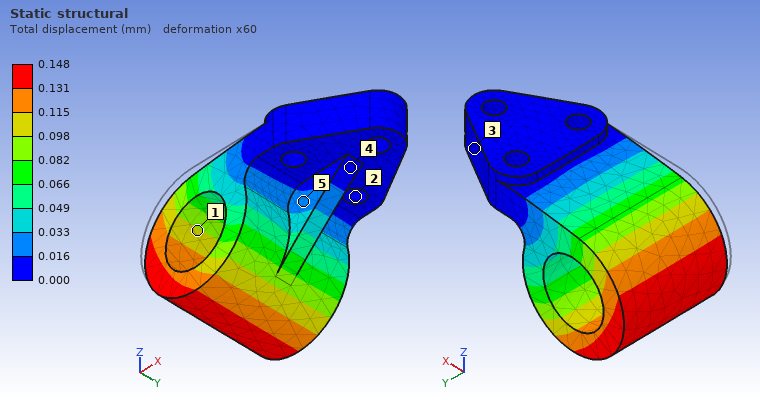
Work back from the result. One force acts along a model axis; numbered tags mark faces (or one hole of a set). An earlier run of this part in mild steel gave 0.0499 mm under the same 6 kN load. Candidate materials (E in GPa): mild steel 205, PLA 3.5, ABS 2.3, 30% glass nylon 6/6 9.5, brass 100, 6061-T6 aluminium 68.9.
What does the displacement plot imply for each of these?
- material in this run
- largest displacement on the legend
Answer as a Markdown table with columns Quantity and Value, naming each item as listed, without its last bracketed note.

| Quantity | Value |
|---|---|
| material in this run | 6061-T6 aluminium |
| largest displacement on the legend | 0.148 mm |
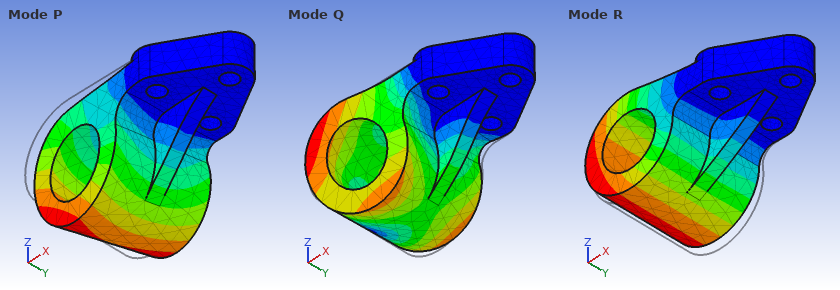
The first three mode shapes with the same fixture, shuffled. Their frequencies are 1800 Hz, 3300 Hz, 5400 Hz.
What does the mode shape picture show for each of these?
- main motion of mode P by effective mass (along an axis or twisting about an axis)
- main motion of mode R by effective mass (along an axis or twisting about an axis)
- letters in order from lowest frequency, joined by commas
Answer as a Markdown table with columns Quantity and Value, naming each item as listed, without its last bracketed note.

| Quantity | Value |
|---|---|
| main motion of mode P by effective mass | along Y |
| main motion of mode R by effective mass | along Z |
| letters in order from lowest frequency, joined by commas | R, P, Q |
